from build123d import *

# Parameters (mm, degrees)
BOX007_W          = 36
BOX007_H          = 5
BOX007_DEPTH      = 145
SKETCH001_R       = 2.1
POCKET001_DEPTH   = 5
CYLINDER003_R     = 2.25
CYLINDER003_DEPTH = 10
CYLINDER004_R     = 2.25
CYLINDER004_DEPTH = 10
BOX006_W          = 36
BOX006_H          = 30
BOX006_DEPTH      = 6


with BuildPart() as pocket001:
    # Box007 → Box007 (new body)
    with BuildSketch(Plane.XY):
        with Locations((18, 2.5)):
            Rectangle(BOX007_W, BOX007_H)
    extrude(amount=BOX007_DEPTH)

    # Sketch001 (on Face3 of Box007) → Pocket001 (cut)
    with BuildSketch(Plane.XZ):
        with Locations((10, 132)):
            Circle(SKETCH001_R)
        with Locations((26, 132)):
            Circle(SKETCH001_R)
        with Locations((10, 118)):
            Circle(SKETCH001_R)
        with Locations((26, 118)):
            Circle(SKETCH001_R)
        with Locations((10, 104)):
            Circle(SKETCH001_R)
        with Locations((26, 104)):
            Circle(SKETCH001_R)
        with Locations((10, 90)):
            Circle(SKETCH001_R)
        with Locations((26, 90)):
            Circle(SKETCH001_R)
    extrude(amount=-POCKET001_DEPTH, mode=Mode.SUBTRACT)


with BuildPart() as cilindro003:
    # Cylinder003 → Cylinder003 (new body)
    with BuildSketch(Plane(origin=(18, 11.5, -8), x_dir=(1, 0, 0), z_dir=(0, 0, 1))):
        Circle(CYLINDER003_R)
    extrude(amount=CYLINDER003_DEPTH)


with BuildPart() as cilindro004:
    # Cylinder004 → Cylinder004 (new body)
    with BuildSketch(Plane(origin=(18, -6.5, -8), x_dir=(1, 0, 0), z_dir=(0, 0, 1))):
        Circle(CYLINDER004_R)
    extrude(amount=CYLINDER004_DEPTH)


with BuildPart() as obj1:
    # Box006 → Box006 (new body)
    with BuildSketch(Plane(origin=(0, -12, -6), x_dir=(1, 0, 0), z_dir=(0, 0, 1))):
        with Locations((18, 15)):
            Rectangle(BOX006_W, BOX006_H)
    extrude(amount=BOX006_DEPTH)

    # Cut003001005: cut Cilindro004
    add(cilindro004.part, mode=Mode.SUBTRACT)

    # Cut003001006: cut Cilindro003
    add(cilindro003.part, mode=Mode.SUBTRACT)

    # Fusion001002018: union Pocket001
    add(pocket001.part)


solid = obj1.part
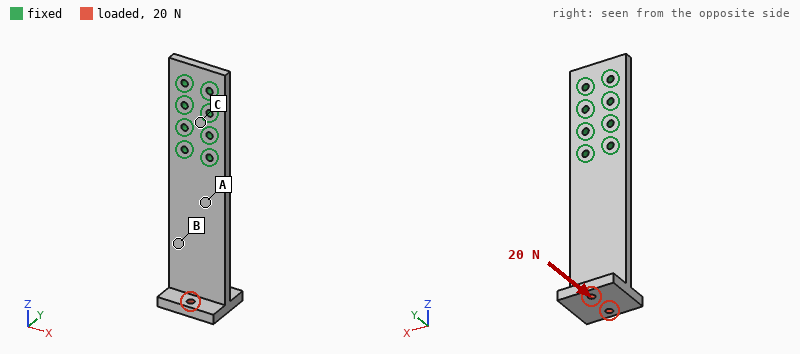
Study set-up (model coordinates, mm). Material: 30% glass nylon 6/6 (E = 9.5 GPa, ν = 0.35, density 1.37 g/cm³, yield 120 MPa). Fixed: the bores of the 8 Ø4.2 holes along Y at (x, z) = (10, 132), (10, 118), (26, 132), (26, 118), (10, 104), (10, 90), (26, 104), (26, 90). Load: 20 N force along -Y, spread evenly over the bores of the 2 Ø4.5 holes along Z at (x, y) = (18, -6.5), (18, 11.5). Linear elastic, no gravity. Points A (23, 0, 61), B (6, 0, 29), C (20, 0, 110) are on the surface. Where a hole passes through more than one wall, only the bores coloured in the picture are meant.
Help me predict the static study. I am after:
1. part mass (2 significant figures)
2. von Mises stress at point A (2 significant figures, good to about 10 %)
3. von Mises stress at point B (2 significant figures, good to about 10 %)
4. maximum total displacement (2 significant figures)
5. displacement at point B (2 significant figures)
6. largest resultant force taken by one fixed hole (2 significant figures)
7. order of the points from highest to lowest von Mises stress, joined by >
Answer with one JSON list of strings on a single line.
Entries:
["44 g", "8.1 MPa", "4.4 MPa", "1.6 mm", "0.72 mm", "28 N", "A > B > C"]
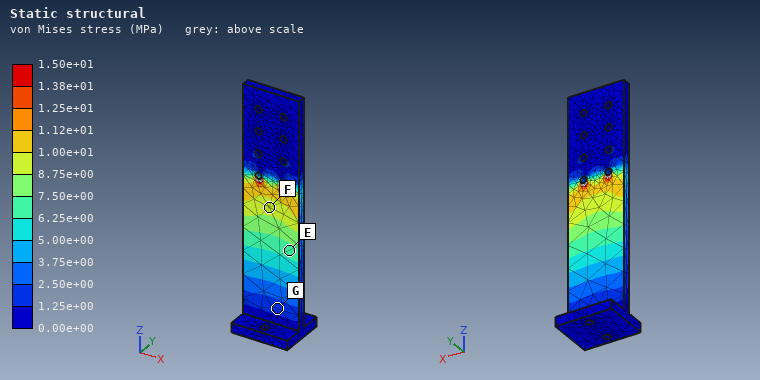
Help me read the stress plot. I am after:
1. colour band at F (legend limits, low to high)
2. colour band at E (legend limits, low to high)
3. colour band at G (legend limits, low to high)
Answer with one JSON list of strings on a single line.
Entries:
["8.75e+00 to 1.00e+01 MPa", "6.25e+00 to 7.50e+00 MPa", "1.25e+00 to 2.50e+00 MPa"]
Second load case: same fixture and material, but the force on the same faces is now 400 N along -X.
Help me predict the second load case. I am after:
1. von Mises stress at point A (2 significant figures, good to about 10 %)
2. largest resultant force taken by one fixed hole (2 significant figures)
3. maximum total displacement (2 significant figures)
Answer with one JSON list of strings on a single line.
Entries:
["8.8 MPa", "1.3 kN", "0.79 mm"]
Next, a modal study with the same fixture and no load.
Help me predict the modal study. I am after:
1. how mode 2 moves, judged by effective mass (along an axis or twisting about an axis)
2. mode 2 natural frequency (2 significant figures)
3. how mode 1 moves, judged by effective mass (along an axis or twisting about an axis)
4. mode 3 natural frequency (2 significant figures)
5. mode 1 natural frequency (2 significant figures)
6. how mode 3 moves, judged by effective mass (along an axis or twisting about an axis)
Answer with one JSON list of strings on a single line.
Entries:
["twisting about Z", "800 Hz", "along Y", "980 Hz", "160 Hz", "along X"]
